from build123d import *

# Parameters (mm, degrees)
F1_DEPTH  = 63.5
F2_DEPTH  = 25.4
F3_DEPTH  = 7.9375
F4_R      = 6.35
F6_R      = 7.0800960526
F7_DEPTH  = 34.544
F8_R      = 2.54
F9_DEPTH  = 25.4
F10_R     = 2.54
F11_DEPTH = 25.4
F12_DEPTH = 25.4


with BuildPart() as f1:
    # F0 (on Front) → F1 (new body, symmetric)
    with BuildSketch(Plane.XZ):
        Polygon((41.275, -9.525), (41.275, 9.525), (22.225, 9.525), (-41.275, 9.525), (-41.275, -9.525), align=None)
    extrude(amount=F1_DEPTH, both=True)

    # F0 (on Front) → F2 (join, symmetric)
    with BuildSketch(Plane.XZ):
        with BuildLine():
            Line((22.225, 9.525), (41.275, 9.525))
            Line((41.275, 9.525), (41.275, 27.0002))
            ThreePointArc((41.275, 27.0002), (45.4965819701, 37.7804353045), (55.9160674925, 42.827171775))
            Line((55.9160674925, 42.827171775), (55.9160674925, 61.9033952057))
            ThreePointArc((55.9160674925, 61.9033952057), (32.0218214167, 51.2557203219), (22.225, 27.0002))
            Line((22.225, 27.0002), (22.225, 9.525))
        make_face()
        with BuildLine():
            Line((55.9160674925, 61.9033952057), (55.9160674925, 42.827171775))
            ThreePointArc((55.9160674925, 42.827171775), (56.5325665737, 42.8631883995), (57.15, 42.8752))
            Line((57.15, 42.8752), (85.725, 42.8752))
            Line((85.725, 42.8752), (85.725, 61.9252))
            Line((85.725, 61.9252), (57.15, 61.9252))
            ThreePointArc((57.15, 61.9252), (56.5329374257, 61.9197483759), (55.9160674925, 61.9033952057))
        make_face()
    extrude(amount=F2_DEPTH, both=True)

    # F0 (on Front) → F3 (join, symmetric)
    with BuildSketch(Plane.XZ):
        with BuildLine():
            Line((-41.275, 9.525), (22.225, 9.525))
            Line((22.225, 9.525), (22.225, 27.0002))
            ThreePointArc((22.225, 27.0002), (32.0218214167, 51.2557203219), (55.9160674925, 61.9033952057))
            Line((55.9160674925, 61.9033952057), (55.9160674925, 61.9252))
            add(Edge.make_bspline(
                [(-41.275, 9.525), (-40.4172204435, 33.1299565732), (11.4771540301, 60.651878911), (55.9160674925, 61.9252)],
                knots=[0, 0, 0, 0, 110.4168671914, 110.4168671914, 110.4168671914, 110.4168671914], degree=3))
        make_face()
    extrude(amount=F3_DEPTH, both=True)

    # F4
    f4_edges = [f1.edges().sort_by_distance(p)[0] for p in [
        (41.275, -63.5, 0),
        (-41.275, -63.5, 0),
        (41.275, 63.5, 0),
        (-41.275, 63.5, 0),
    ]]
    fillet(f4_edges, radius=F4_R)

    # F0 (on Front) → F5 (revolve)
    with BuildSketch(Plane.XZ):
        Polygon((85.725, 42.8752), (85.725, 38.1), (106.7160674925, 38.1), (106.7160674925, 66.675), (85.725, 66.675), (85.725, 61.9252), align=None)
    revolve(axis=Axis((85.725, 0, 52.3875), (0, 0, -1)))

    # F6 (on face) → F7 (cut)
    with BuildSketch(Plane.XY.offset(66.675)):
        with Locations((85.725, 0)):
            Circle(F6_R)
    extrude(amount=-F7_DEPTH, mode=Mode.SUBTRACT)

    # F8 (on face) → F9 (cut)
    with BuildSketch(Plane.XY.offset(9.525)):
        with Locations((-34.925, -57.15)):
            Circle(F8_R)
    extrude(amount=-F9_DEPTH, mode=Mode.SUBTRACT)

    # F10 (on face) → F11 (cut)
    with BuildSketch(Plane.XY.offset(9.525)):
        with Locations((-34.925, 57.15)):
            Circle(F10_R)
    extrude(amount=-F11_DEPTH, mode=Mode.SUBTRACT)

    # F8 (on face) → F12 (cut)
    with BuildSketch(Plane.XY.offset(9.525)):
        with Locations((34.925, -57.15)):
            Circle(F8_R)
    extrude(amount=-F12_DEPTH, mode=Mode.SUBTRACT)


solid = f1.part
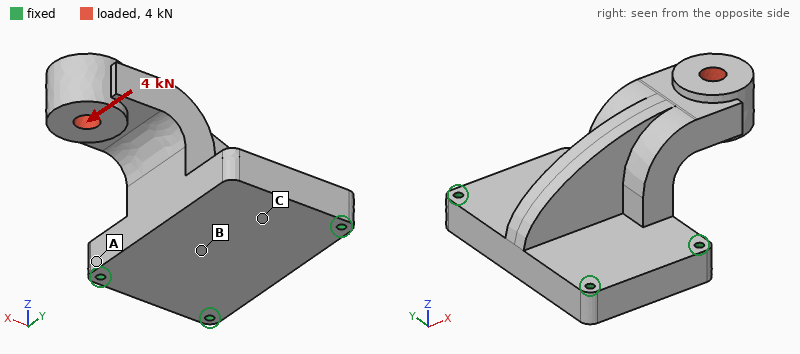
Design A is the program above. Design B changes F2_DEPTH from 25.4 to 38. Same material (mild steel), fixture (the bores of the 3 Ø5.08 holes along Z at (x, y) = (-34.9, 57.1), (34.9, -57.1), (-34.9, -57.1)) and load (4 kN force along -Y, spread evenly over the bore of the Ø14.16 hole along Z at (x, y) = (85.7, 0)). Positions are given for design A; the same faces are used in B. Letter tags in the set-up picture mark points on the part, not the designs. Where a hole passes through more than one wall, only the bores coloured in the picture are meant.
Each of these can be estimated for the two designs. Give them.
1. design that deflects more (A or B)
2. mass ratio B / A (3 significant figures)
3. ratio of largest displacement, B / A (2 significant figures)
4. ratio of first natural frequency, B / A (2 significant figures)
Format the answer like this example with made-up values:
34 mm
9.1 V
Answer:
A
1.12
0.58
0.96
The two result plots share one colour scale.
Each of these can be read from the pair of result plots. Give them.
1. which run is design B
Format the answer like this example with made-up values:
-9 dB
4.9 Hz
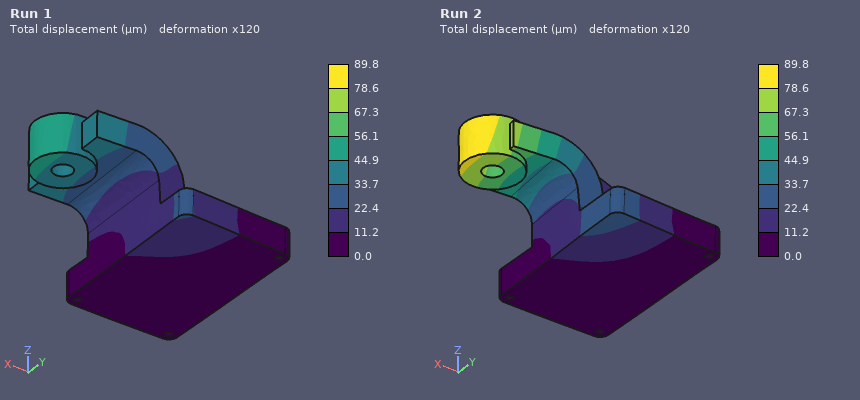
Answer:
Run 1
